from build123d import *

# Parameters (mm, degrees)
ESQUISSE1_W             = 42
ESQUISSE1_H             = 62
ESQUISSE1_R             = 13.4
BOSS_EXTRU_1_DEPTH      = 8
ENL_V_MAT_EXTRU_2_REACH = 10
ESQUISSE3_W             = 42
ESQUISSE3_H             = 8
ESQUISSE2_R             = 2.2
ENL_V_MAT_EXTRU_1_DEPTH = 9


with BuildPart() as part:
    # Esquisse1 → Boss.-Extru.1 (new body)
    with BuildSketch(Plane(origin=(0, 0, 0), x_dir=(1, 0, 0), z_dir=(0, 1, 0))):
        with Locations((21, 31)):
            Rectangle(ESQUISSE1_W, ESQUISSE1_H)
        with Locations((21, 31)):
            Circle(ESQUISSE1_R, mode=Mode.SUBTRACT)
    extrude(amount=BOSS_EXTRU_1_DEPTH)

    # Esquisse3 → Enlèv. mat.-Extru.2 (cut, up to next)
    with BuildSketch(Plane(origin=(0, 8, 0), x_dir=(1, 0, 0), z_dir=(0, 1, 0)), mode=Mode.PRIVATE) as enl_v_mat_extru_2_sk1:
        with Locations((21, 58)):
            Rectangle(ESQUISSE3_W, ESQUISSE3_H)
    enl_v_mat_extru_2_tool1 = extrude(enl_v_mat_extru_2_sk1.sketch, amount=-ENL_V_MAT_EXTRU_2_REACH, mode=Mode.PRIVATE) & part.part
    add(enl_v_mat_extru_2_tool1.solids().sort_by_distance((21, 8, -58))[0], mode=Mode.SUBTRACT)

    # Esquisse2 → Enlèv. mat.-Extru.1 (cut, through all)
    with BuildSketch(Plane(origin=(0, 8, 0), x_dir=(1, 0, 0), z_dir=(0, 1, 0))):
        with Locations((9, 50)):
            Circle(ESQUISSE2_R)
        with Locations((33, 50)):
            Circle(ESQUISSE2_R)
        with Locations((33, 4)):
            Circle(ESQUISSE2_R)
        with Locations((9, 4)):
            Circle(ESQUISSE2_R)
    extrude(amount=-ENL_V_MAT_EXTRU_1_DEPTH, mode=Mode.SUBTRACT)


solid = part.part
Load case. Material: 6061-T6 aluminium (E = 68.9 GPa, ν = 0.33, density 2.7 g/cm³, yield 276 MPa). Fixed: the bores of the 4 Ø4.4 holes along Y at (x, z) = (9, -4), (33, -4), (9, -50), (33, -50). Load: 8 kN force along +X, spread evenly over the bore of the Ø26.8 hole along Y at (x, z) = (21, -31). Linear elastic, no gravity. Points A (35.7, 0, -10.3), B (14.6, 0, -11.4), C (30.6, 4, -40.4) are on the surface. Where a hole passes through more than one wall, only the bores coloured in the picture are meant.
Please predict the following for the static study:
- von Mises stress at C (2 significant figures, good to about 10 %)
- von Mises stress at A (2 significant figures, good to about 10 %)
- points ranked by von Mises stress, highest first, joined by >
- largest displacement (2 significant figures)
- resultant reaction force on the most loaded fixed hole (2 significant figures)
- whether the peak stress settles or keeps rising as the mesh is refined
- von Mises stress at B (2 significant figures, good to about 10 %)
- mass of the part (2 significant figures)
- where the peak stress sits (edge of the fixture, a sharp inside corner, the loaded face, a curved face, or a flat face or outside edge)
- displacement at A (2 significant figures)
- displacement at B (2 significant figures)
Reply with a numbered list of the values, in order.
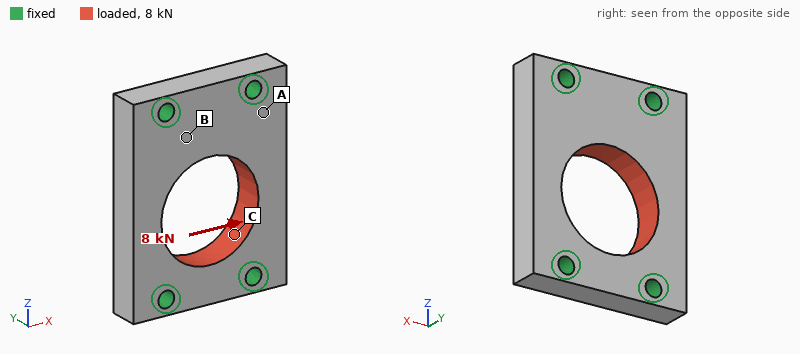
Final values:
1. 47 MPa
2. 12 MPa
3. C > B > A
4. 17 µm
5. 2.1 kN
6. keeps rising
7. 29 MPa
8. 35 g
9. edge of the fixture
10. 4.2 µm
11. 4.8 µm
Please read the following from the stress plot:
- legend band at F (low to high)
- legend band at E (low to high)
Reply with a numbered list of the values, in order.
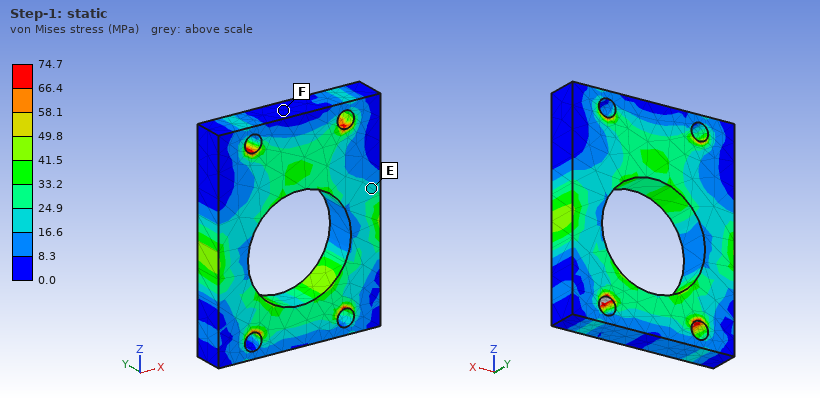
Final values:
1. 0.0 to 8.3 MPa
2. 16.6 to 24.9 MPa
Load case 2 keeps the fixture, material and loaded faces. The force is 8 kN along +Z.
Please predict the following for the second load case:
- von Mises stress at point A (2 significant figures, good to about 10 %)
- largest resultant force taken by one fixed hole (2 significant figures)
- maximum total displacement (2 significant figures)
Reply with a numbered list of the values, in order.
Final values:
1. 14 MPa
2. 2.2 kN
3. 4.9 µm
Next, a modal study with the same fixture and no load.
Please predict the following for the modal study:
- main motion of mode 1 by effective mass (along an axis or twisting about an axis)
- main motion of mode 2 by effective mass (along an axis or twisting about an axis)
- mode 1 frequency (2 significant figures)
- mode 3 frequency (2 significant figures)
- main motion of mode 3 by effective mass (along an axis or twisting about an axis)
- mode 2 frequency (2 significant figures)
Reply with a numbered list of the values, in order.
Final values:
1. along Y
2. twisting about Z
3. 17 kHz
4. 30 kHz
5. along X
6. 18 kHz
